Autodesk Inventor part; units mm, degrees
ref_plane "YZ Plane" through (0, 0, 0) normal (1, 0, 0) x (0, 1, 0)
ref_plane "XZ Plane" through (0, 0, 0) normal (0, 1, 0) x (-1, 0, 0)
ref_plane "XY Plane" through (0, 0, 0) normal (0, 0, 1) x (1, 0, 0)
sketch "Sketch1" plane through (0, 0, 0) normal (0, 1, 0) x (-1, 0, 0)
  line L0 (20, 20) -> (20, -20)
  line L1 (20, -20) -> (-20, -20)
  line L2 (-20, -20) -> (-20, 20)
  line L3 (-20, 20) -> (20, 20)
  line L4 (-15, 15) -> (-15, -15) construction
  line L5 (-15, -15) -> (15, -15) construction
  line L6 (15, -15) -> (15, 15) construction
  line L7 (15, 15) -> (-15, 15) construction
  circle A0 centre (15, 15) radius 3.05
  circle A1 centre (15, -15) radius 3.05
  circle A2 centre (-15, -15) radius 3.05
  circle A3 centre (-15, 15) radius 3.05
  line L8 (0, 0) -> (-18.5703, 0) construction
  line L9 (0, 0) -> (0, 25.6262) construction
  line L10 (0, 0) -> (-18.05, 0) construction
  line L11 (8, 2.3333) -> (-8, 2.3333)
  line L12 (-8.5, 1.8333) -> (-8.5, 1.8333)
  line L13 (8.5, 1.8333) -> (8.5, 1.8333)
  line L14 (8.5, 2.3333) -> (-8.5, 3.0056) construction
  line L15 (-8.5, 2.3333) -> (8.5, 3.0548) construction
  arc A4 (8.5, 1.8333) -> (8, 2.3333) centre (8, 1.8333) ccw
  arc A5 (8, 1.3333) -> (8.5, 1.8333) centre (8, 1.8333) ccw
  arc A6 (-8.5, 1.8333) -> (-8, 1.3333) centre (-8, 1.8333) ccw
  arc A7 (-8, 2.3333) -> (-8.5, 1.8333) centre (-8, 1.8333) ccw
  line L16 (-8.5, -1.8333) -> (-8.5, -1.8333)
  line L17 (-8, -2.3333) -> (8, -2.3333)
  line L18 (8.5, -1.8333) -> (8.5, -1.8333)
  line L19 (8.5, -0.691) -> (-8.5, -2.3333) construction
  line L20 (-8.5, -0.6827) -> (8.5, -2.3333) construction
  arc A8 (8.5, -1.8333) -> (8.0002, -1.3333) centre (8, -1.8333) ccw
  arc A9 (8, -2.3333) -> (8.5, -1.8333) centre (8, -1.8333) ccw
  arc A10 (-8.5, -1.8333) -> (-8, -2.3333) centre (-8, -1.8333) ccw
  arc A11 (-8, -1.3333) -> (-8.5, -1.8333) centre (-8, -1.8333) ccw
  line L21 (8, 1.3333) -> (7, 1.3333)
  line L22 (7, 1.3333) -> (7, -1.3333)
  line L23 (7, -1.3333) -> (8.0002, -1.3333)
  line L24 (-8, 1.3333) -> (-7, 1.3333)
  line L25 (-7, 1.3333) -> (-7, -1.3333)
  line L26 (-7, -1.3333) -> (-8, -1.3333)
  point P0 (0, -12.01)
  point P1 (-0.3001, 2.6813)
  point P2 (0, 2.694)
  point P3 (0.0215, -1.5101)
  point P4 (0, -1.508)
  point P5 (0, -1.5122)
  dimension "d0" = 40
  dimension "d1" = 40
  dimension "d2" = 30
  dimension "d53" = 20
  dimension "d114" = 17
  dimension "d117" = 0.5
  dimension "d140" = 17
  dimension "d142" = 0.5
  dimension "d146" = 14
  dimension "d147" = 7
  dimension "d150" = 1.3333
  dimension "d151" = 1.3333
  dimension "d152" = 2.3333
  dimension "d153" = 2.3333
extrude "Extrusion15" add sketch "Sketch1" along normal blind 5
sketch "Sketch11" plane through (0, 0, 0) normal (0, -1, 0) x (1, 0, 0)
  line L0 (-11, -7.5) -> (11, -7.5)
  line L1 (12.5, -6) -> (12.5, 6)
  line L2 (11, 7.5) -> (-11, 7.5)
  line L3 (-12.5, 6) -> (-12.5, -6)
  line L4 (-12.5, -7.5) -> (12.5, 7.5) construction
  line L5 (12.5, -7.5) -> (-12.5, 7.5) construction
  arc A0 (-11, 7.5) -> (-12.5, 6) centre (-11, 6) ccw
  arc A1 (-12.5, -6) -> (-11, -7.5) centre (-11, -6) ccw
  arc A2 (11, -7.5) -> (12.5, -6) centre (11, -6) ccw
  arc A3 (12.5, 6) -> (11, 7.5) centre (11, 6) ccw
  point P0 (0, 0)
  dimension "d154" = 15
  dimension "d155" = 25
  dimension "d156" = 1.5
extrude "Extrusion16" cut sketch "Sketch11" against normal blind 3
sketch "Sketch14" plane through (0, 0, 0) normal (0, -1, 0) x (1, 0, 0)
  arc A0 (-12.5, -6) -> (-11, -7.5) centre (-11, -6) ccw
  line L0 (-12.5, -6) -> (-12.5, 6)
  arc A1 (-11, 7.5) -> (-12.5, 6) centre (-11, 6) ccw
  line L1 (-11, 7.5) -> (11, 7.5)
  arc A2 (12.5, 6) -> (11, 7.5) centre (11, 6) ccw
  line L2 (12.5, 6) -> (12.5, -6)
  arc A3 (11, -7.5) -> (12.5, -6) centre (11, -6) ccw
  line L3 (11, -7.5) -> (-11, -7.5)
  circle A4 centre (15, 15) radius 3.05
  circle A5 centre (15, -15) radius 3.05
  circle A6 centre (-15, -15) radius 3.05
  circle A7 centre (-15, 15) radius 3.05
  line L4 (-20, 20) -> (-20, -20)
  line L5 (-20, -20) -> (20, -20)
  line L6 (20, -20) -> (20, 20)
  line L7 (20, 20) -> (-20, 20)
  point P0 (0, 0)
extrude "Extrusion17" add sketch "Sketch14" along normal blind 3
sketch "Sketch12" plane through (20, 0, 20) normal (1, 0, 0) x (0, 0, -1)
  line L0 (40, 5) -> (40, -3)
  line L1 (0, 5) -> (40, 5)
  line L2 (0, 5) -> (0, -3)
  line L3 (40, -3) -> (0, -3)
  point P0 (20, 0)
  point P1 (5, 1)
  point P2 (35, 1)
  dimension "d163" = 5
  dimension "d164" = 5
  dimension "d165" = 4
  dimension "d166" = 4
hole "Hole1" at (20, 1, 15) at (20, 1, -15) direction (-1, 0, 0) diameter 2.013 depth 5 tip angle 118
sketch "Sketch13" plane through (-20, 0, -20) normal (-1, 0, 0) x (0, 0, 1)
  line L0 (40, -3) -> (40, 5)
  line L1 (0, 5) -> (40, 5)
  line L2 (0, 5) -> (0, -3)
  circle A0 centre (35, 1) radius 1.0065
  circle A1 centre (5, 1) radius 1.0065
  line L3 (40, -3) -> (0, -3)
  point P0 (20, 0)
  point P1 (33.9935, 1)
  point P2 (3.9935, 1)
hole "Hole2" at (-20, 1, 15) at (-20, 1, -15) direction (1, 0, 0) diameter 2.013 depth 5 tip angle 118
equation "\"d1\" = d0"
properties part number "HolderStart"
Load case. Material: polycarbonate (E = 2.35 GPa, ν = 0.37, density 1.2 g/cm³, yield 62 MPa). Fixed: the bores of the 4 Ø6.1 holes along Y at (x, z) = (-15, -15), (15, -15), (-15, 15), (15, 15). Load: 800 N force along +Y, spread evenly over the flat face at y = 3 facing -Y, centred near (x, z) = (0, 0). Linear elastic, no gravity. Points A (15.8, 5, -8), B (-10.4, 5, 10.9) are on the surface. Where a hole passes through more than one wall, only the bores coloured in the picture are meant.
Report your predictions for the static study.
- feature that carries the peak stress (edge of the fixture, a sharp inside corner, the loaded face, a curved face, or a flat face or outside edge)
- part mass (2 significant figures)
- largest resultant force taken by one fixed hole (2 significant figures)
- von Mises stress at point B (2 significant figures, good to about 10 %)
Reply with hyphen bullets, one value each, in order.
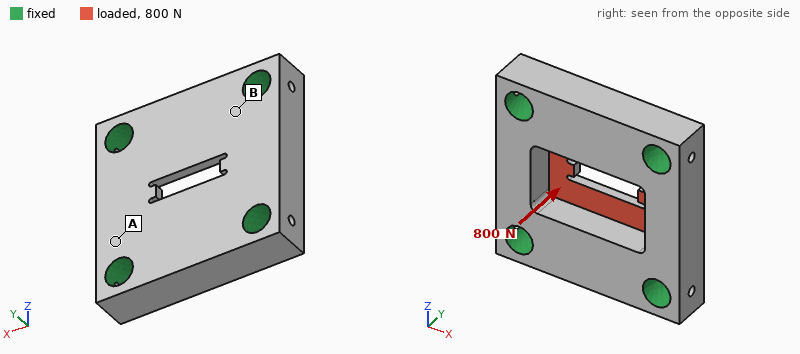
- a curved face
- 11 g
- 210 N
- 9.5 MPa
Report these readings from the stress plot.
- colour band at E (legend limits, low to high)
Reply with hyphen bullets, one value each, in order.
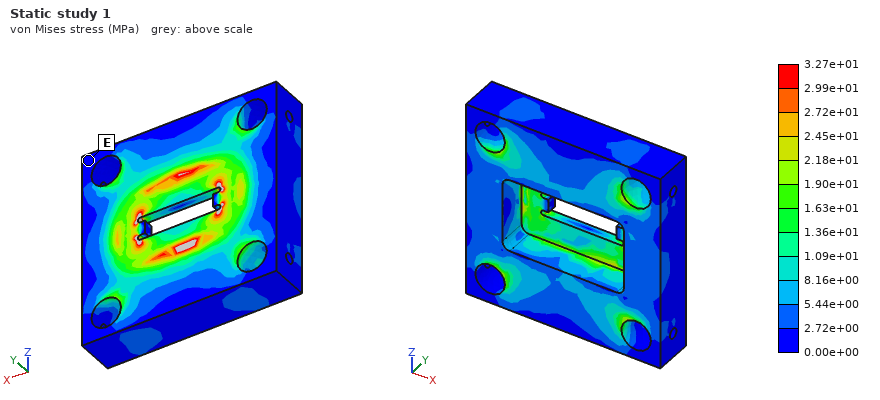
- 0.00e+00 to 2.72e+00 MPa
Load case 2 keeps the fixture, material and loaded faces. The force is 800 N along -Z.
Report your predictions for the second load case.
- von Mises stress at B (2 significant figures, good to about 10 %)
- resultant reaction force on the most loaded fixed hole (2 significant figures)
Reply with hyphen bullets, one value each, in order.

- 6.5 MPa
- 210 N
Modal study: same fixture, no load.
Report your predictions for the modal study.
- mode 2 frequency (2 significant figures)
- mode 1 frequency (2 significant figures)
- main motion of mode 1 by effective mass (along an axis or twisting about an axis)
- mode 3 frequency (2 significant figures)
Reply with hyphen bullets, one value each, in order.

- 9700 Hz
- 8900 Hz
- along Y
- 12 kHz
